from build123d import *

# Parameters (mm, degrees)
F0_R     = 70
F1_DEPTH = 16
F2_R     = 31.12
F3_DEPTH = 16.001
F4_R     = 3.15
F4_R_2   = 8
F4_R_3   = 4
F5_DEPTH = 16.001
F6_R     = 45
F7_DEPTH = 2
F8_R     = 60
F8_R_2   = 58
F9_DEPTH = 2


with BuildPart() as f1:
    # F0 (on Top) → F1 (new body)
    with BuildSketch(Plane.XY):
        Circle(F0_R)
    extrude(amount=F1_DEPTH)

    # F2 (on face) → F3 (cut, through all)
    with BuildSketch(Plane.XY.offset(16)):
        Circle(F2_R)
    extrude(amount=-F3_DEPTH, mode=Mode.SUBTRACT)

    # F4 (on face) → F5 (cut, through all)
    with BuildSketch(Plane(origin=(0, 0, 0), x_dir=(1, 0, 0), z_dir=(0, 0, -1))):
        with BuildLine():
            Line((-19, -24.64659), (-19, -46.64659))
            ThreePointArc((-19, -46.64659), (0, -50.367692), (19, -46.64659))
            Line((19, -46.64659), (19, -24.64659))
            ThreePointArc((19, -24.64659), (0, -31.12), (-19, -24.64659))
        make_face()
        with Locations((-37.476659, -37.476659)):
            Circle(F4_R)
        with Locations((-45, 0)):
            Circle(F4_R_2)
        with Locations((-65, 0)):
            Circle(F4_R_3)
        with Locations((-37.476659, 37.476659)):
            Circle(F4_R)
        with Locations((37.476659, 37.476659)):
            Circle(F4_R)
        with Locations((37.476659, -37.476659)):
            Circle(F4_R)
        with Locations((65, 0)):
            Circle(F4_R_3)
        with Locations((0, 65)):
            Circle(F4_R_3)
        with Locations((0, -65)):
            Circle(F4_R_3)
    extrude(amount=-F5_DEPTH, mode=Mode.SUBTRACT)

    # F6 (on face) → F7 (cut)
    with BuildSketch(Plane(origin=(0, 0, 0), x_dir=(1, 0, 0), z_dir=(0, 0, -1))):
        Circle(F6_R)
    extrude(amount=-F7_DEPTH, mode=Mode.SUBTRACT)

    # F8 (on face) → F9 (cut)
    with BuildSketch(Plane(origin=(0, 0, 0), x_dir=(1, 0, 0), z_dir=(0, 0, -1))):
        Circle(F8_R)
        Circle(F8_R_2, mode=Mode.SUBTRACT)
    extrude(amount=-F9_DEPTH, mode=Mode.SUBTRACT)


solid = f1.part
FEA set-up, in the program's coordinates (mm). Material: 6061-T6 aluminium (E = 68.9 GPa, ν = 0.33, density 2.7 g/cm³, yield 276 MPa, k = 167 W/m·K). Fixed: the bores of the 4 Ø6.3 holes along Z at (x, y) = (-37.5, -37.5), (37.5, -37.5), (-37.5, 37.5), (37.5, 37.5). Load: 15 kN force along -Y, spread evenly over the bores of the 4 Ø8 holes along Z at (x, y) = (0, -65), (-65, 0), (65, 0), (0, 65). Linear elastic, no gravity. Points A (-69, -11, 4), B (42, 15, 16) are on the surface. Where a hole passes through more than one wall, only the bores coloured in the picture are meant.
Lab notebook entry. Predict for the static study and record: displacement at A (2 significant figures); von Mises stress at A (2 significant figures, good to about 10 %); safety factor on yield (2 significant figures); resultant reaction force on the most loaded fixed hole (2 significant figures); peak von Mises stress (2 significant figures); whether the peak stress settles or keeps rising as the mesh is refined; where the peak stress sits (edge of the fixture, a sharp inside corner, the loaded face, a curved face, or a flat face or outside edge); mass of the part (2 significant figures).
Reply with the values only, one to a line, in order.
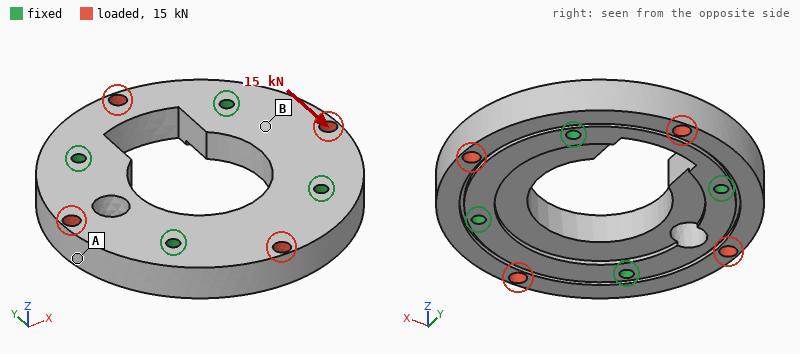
5.8 µm
12 MPa
3.3
4.4 kN
83 MPa
settles
a curved face
460 g
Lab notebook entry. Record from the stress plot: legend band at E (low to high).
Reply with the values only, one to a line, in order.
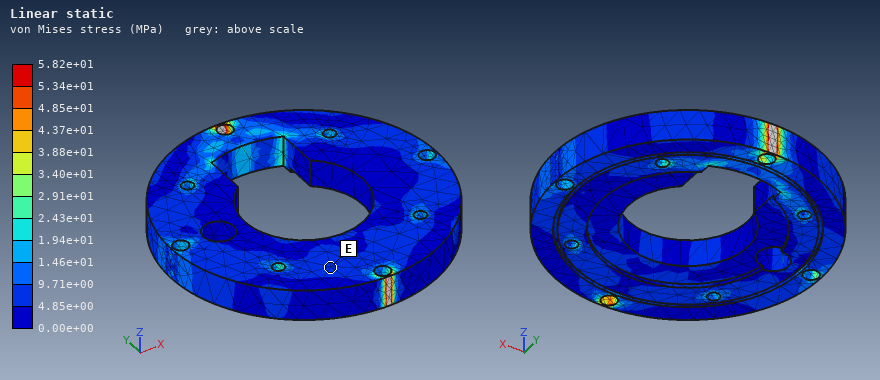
4.85e+00 to 9.71e+00 MPa
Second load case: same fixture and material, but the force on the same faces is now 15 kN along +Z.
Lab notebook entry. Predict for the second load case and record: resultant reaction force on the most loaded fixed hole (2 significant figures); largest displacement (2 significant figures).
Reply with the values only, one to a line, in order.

3.8 kN
82 µm
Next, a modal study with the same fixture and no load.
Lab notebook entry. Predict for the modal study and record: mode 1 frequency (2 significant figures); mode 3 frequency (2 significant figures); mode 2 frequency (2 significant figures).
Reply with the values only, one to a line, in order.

6900 Hz
7700 Hz
7700 Hz
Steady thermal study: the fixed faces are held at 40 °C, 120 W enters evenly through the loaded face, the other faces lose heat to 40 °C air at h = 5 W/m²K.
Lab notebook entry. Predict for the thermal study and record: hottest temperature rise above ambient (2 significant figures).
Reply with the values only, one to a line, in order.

16 K
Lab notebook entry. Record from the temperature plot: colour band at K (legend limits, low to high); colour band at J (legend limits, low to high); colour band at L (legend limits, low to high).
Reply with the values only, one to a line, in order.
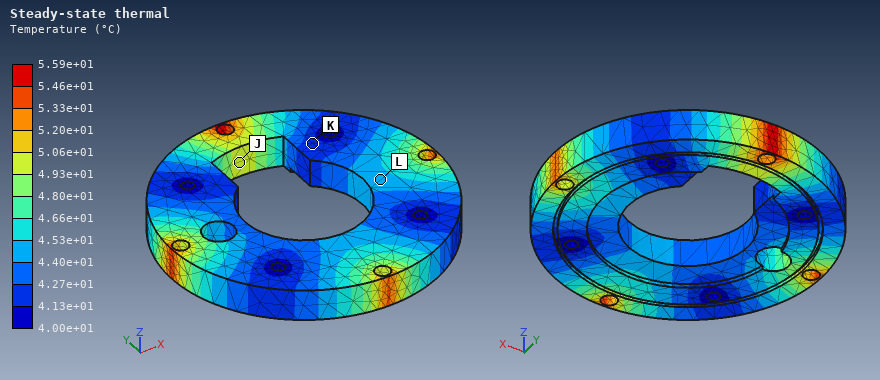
4.13e+01 to 4.27e+01 °C
4.93e+01 to 5.06e+01 °C
4.40e+01 to 4.53e+01 °C
